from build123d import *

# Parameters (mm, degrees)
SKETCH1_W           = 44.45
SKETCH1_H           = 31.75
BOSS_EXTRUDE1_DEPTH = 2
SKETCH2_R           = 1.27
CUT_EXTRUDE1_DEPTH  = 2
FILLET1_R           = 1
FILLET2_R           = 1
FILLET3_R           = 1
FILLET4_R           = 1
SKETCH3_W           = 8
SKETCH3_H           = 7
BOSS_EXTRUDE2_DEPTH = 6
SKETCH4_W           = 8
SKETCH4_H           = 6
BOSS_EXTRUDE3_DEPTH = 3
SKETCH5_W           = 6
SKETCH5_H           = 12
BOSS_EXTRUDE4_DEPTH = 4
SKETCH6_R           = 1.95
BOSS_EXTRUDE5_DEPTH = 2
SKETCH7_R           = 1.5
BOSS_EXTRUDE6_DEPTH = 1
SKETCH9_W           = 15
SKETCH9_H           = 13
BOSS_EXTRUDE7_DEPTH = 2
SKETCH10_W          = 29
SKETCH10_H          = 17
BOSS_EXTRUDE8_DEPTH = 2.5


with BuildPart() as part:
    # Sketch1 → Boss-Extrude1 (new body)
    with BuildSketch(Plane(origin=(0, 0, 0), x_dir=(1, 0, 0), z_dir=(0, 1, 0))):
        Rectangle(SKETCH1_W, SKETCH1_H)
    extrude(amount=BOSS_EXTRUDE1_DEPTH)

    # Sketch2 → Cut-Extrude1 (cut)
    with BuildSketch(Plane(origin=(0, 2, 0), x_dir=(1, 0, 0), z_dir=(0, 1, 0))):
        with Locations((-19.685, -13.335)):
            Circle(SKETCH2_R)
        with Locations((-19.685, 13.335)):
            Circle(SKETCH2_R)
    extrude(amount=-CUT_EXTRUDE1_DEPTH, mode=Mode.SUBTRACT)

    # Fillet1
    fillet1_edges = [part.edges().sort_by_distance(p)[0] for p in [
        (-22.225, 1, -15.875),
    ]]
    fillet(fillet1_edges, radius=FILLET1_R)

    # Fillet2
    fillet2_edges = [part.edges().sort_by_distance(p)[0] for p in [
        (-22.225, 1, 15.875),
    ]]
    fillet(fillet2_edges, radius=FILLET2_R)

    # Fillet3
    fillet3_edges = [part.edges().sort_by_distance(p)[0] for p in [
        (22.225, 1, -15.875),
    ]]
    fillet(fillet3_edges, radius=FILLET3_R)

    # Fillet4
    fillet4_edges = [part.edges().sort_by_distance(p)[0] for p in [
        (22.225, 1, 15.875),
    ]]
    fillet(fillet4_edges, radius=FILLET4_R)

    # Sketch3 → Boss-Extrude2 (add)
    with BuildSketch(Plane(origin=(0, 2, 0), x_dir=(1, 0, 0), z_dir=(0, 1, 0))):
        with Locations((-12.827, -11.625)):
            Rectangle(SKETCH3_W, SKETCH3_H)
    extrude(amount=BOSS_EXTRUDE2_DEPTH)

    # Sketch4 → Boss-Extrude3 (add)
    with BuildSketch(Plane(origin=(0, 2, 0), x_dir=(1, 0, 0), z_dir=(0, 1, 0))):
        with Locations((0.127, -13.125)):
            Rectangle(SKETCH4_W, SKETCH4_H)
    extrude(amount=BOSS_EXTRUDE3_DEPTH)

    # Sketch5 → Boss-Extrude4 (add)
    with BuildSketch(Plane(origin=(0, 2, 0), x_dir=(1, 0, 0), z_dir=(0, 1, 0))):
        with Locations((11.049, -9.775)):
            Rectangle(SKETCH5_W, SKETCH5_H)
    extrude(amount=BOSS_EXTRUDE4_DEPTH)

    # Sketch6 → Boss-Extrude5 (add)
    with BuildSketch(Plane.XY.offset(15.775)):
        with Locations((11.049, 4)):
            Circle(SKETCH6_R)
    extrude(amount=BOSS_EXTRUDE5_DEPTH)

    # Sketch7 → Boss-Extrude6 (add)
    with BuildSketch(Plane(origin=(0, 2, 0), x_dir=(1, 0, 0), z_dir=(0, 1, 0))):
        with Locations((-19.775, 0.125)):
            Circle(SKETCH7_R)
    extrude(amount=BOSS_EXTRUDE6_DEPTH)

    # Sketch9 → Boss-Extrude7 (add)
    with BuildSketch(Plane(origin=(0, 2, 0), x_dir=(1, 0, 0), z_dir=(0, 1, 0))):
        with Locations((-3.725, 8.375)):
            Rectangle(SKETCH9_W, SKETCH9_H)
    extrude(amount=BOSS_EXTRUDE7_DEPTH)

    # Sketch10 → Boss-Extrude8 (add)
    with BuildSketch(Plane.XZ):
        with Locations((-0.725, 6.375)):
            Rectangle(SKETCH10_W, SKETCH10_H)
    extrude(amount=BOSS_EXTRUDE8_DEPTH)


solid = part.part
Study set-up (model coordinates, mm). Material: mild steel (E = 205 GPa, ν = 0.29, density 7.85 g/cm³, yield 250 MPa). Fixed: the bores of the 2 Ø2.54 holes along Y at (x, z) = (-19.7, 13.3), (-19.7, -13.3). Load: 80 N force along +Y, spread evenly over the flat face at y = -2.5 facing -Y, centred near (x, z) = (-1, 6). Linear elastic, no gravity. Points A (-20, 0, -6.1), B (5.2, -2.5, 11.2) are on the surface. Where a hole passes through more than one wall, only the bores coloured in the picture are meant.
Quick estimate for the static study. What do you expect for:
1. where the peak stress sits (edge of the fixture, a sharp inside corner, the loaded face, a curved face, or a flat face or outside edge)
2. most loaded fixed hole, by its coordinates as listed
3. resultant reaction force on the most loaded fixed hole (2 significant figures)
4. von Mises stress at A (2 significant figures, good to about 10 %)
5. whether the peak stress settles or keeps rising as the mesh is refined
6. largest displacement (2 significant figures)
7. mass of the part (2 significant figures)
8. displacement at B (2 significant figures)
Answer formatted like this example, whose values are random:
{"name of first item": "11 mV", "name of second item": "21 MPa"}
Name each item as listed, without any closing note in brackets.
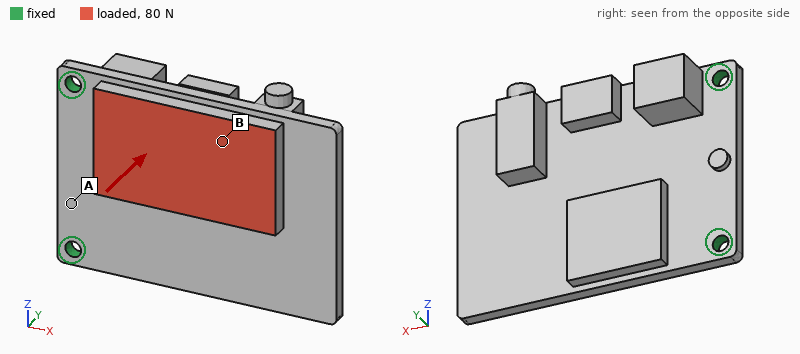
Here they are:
{"where the peak stress sits": "edge of the fixture", "most loaded fixed hole, by its coordinates as listed": "(-19.7, 13.3)", "resultant reaction force on the most loaded fixed hole": "55 N", "von Mises stress at A": "35 MPa", "whether the peak stress settles or keeps rising as the mesh is refined": "keeps rising", "largest displacement": "96 µm", "mass of the part": "41 g", "displacement at B": "55 µm"}
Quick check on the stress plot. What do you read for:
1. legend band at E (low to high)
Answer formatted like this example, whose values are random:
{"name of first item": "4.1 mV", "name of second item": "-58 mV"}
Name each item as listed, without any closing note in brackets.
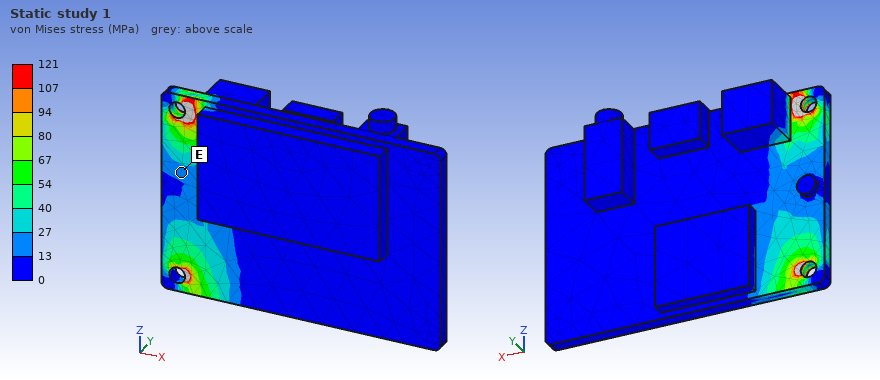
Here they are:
{"legend band at E": "13 to 27 MPa"}
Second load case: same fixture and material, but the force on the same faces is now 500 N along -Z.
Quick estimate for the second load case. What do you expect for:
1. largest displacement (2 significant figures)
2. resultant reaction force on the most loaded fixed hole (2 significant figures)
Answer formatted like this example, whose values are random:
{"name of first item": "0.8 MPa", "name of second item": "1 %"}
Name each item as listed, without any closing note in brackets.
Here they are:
{"largest displacement": "11 µm", "resultant reaction force on the most loaded fixed hole": "440 N"}
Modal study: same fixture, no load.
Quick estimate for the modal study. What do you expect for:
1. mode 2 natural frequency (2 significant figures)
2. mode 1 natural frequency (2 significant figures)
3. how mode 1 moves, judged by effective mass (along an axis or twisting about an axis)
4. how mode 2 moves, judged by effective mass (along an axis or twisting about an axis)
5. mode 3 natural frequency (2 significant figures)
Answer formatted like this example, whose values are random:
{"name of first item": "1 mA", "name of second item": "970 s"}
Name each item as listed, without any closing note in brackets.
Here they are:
{"mode 2 natural frequency": "5000 Hz", "mode 1 natural frequency": "920 Hz", "how mode 1 moves, judged by effective mass": "along Y", "how mode 2 moves, judged by effective mass": "twisting about X", "mode 3 natural frequency": "8300 Hz"}
